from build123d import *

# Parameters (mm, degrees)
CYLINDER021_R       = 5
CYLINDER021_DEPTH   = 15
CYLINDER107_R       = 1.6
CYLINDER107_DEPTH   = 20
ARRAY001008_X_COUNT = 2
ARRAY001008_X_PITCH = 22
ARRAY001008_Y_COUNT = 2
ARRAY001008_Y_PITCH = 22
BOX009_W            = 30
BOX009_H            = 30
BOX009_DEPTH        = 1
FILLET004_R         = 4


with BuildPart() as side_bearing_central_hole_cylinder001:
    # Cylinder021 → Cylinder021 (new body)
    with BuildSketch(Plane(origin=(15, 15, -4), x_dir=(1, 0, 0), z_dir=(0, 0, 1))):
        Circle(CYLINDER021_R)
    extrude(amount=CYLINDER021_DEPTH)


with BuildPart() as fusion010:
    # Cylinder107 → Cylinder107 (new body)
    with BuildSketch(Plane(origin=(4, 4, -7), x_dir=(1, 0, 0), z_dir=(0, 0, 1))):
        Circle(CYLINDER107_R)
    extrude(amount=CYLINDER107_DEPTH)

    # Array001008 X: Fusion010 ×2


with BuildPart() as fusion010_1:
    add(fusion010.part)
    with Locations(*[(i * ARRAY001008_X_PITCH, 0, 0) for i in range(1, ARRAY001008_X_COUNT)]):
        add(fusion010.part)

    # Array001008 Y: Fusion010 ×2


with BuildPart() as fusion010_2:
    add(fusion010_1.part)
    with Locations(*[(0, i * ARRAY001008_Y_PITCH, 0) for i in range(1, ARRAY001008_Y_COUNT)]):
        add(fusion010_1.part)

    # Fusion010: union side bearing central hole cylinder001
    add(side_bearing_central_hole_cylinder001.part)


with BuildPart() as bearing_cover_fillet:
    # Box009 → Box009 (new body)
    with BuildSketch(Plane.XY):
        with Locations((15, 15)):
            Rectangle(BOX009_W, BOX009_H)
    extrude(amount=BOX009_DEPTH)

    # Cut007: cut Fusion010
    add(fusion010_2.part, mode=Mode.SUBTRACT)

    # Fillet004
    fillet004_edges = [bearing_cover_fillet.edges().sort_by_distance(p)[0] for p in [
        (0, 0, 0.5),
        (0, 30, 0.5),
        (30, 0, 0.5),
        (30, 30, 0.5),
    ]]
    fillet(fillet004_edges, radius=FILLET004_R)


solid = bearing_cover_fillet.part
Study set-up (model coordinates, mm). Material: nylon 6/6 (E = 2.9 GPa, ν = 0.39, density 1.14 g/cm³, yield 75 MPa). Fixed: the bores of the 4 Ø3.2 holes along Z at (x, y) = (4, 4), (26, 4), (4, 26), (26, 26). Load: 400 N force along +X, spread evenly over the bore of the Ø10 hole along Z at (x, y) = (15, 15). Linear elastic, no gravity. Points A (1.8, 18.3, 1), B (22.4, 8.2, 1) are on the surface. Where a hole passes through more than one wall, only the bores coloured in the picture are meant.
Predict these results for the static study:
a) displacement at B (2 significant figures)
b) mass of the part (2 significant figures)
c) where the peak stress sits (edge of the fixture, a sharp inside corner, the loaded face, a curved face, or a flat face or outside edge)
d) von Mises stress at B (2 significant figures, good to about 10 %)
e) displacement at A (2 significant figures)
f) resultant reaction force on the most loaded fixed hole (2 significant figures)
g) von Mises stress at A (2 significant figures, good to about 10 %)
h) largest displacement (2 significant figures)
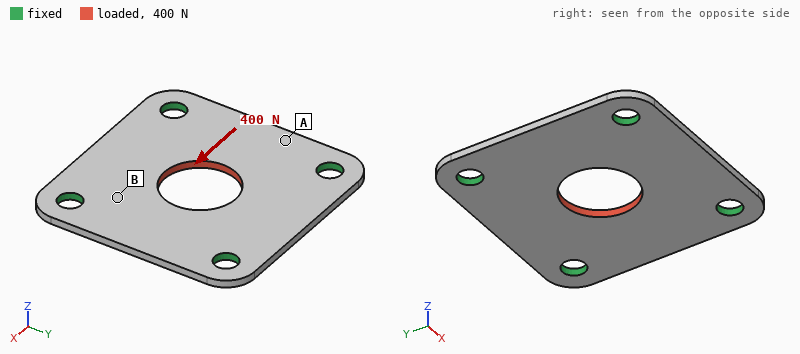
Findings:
33 µm
0.88 g
edge of the fixture
14 MPa
52 µm
110 N
5.8 MPa
77 µm
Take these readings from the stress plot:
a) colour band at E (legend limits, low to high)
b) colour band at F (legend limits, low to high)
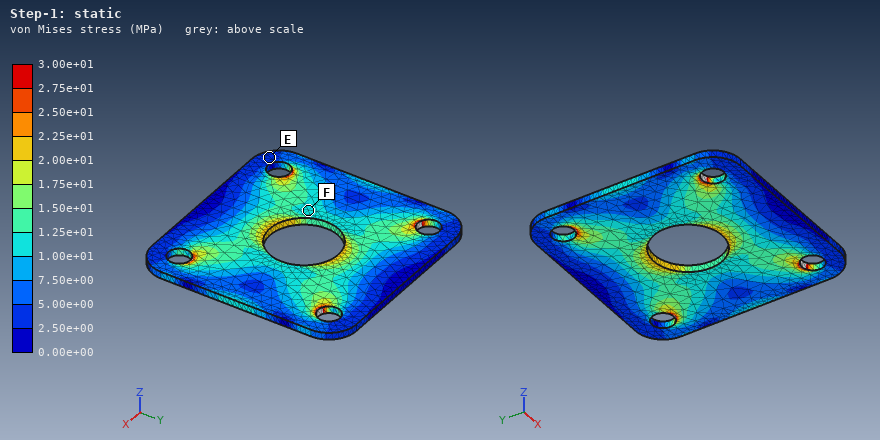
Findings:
2.50e+00 to 5.00e+00 MPa
1.00e+01 to 1.25e+01 MPa
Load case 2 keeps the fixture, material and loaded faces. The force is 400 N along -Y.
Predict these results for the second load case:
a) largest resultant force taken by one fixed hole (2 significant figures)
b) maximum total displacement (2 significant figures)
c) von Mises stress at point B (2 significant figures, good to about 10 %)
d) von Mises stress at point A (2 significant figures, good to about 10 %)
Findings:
110 N
77 µm
14 MPa
3.1 MPa
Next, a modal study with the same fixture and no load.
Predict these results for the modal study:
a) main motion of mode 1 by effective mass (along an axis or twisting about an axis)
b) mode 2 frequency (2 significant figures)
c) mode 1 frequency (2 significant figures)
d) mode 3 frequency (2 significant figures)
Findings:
along Z
4400 Hz
3200 Hz
4400 Hz
